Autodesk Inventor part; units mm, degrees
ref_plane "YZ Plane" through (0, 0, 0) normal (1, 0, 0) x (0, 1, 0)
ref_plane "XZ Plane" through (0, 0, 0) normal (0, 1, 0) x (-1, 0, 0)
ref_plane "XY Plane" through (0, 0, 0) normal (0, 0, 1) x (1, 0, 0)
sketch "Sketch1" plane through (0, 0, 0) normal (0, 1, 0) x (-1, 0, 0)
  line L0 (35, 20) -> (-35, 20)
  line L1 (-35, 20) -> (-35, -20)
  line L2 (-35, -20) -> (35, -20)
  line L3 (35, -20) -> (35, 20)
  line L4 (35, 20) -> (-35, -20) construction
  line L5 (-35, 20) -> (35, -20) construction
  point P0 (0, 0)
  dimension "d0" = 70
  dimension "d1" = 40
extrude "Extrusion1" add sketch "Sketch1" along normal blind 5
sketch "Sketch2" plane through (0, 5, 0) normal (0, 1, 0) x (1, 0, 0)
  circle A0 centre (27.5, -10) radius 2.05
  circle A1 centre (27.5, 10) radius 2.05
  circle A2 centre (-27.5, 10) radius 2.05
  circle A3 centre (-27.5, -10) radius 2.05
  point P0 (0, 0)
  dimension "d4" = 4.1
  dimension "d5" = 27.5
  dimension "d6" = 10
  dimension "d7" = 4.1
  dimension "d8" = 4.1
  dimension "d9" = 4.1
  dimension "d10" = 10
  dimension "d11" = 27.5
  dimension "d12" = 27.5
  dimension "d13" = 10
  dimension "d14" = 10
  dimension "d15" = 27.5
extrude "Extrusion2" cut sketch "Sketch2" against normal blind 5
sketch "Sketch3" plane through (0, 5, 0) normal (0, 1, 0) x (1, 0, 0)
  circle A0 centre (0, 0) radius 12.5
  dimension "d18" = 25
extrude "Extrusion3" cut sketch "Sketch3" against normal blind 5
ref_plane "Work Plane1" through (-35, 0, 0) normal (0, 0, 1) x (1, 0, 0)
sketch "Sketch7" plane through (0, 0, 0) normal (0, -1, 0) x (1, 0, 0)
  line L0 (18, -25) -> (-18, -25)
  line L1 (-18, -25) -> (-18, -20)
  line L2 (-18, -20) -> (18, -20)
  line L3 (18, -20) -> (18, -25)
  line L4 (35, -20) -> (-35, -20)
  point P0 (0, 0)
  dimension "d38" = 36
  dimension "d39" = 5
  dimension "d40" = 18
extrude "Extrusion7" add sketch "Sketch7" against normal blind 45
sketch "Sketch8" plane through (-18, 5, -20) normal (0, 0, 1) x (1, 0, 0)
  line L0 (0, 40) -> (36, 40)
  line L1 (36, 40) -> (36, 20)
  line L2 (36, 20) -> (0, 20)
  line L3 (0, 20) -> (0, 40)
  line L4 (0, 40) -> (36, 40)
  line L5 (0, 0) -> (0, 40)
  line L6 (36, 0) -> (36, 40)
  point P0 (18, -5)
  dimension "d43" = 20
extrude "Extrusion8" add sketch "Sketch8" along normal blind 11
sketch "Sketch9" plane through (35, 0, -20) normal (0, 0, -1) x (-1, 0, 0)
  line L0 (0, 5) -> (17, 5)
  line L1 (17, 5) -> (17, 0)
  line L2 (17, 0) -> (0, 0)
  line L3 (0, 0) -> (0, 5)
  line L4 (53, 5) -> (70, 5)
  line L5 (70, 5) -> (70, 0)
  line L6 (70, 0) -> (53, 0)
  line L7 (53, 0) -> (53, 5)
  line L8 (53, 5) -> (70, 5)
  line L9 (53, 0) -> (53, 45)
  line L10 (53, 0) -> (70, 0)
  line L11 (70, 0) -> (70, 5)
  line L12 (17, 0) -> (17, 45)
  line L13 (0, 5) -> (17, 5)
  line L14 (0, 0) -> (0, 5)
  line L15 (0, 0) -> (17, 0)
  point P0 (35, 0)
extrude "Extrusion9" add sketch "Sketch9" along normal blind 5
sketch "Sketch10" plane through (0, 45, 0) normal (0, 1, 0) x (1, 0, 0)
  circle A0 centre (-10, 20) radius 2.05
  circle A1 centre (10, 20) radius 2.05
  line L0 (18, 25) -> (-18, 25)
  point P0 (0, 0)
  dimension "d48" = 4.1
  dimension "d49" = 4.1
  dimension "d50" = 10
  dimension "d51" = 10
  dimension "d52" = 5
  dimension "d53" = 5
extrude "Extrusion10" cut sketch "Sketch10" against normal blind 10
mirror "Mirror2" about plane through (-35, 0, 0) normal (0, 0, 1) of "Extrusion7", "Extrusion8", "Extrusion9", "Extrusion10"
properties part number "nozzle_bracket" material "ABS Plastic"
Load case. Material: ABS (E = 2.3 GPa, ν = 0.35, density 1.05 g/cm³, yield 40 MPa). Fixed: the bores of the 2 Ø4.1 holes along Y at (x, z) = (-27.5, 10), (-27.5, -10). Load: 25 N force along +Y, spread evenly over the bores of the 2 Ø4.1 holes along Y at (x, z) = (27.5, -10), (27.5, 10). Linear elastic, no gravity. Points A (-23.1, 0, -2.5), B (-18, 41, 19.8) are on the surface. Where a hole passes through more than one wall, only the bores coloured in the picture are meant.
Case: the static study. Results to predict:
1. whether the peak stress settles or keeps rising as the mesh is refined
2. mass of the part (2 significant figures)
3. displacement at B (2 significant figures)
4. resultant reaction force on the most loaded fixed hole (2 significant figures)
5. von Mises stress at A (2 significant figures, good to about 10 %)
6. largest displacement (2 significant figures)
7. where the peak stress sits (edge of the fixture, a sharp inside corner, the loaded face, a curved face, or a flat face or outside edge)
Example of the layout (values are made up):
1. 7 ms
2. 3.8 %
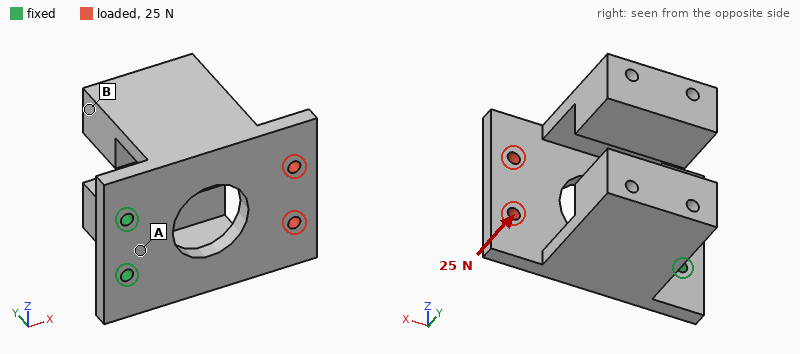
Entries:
1. keeps rising
2. 47 g
3. 0.72 mm
4. 14 N
5. 4.0 MPa
6. 1.1 mm
7. edge of the fixture
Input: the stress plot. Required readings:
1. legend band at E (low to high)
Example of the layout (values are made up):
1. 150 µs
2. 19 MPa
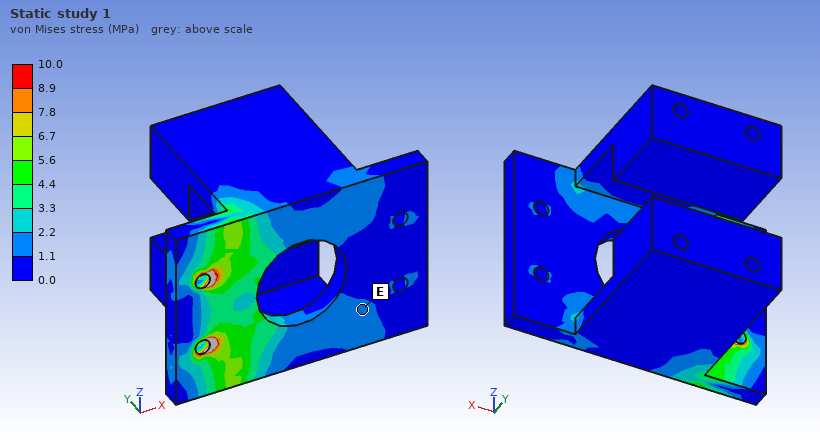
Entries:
1. 1.1 to 2.2 MPa
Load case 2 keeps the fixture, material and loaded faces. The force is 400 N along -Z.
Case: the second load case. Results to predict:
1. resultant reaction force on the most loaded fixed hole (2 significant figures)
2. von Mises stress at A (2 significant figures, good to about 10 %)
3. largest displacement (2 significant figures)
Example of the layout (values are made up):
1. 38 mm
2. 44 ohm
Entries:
1. 940 N
2. 14 MPa
3. 1.0 mm
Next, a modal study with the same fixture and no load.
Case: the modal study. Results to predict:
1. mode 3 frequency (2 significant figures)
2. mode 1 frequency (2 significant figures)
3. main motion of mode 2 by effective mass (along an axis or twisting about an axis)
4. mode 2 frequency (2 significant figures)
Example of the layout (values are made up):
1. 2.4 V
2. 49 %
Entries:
1. 250 Hz
2. 170 Hz
3. along Z
4. 200 Hz
